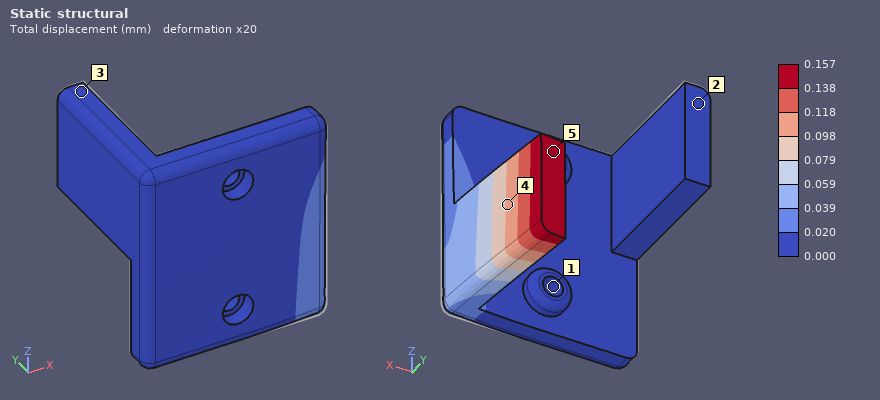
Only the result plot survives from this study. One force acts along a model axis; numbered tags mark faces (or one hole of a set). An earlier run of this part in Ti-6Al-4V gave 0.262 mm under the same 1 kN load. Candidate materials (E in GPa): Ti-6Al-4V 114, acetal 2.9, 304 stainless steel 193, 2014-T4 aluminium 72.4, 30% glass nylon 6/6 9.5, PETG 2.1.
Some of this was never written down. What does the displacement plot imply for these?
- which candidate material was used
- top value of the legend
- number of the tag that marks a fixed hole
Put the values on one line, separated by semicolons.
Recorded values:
304 stainless steel; 0.157 mm; 1
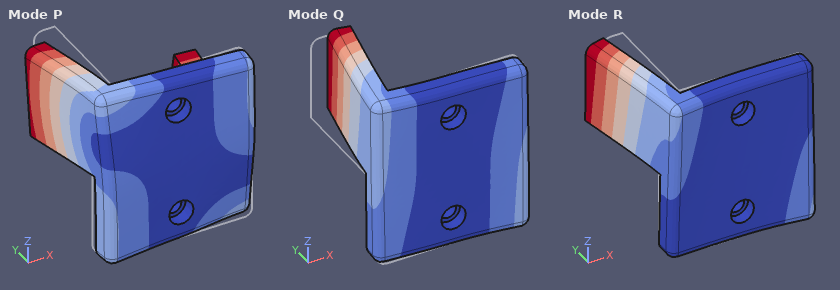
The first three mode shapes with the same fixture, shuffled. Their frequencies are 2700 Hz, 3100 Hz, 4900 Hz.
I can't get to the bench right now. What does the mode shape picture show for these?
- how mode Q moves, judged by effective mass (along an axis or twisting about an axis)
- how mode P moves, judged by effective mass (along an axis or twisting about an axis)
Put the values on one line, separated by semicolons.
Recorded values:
along X; twisting about Y
